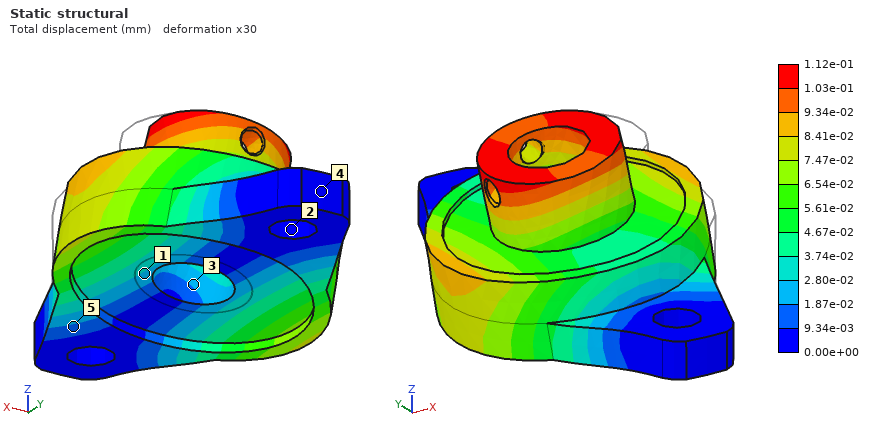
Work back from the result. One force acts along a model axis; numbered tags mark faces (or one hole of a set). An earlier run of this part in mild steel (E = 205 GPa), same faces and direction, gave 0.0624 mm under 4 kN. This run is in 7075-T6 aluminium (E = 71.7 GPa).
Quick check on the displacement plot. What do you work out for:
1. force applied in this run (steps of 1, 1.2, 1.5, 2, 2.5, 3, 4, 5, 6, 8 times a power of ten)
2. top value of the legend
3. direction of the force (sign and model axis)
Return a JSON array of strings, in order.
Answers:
["2.5 kN", "1.12e-01 mm", "-X"]
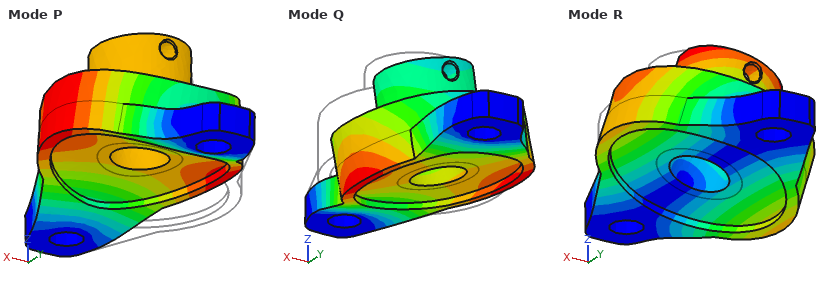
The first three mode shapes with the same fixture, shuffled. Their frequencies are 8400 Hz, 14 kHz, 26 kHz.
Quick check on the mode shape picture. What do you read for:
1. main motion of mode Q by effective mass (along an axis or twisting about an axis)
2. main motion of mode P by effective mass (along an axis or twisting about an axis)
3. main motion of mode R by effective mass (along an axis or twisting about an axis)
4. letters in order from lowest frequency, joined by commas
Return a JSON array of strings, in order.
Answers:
["along X", "along Z", "along X", "R, P, Q"]
